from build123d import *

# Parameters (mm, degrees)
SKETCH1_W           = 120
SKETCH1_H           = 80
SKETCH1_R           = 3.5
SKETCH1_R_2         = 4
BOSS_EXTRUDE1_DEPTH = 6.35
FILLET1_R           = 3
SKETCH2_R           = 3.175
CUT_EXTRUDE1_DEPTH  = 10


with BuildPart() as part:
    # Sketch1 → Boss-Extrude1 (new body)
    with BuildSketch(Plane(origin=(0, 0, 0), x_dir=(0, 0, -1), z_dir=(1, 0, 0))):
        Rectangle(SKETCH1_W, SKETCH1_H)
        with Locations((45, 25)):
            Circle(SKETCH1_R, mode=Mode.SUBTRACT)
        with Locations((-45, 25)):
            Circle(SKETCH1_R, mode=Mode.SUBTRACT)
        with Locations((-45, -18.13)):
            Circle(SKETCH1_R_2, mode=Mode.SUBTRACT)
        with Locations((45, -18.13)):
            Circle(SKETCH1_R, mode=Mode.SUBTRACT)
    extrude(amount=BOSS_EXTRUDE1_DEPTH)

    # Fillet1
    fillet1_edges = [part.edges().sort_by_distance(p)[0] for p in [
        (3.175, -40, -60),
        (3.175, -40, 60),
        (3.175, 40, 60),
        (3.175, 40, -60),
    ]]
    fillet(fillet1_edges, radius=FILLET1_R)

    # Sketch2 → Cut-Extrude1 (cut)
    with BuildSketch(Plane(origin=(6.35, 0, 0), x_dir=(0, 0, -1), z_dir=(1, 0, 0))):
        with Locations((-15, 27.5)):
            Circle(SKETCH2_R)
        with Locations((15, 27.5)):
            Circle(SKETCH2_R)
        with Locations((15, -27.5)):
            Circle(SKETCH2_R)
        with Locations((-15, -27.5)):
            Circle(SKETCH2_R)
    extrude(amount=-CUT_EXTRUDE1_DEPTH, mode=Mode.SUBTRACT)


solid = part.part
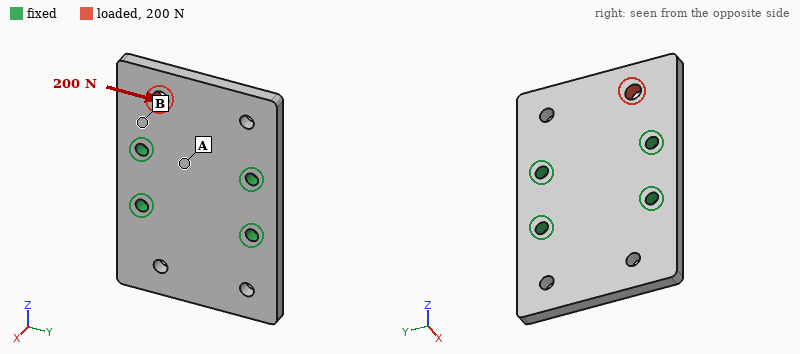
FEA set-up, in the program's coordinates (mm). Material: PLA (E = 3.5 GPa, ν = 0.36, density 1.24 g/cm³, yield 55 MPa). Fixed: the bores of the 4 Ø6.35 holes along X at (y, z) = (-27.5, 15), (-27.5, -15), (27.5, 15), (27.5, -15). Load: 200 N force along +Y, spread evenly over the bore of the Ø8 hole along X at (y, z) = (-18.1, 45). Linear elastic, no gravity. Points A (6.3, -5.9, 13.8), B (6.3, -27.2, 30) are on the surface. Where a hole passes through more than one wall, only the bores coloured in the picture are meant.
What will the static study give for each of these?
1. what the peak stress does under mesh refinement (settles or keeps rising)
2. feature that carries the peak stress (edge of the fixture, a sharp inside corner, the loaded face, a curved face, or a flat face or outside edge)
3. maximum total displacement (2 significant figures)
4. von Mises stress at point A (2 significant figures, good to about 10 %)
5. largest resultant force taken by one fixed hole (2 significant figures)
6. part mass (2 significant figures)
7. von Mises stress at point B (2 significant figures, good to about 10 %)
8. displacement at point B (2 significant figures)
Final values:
keeps rising
edge of the fixture
21 µm
0.37 MPa
130 N
73 g
0.86 MPa
8.5 µm
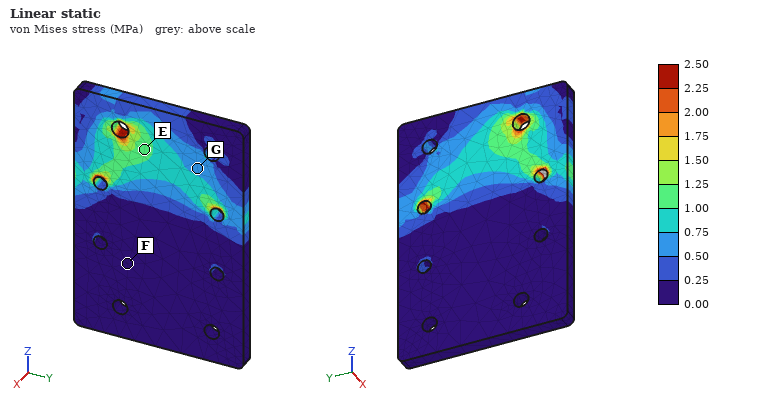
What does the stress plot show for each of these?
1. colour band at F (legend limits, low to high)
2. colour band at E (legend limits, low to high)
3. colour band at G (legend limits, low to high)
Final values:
0.00 to 0.25 MPa
1.00 to 1.25 MPa
0.50 to 0.75 MPa
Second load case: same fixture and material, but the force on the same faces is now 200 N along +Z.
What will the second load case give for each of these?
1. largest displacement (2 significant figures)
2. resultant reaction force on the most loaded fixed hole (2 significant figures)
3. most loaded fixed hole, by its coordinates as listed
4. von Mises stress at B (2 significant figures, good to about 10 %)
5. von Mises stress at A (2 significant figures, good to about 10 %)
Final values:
13 µm
130 N
(-27.5, 15)
1.1 MPa
0.31 MPa
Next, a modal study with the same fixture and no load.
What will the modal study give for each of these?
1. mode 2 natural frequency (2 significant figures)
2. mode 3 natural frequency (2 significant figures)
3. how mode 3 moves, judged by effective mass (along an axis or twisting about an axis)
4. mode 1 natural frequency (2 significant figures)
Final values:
820 Hz
1400 Hz
twisting about Z
810 Hz
